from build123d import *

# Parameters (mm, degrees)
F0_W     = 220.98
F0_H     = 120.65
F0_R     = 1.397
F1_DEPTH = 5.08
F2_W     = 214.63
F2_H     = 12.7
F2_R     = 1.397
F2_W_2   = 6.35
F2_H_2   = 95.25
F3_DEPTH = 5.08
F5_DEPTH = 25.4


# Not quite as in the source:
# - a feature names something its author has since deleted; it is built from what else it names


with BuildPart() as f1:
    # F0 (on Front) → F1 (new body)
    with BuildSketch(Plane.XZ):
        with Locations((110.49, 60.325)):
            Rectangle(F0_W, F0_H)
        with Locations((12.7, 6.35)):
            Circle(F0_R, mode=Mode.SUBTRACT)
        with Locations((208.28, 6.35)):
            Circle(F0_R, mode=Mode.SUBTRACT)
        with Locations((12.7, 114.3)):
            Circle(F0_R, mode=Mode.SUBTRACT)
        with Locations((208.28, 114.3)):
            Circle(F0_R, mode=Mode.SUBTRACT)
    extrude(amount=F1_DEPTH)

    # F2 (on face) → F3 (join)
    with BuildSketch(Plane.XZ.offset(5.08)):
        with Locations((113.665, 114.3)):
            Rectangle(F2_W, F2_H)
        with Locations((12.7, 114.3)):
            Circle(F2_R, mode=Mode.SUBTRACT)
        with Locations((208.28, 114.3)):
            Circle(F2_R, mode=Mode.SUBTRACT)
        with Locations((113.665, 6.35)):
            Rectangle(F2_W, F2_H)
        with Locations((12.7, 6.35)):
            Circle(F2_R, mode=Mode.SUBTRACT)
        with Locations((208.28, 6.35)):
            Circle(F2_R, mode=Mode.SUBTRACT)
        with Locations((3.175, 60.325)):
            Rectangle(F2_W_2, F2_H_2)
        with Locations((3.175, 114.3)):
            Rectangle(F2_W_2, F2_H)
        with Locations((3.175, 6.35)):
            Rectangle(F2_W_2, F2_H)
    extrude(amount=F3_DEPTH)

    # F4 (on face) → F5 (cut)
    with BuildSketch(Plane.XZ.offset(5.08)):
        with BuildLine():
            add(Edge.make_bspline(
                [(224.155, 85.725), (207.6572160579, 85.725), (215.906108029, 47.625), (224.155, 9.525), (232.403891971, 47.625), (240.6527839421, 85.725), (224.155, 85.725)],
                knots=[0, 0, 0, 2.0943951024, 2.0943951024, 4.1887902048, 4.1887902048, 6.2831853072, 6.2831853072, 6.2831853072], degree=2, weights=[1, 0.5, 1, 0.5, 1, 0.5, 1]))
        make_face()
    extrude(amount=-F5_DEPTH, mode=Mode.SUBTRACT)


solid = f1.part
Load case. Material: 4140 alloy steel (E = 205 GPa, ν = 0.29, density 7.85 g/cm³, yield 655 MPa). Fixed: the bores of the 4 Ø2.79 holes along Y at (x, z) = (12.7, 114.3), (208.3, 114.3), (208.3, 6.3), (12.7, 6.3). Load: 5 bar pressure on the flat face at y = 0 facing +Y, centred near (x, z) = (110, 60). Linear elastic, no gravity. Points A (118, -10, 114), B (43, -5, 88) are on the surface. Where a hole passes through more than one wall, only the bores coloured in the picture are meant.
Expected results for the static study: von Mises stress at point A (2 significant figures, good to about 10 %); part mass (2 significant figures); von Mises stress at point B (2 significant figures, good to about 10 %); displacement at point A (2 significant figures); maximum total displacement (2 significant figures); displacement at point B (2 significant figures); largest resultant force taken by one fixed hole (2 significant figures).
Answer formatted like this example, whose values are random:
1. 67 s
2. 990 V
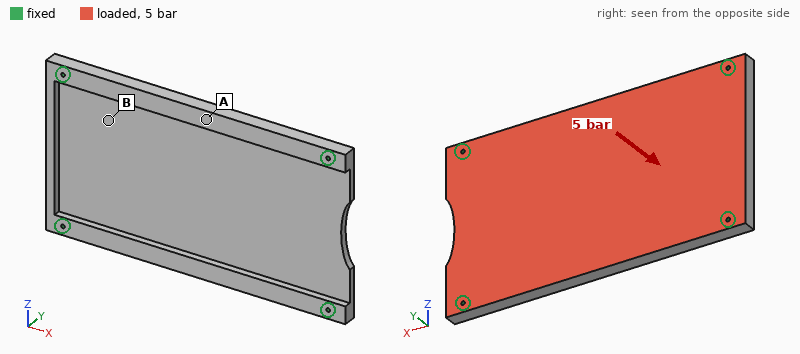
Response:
1. 160 MPa
2. 1.3 kg
3. 37 MPa
4. 0.34 mm
5. 0.48 mm
6. 0.18 mm
7. 5.0 kN
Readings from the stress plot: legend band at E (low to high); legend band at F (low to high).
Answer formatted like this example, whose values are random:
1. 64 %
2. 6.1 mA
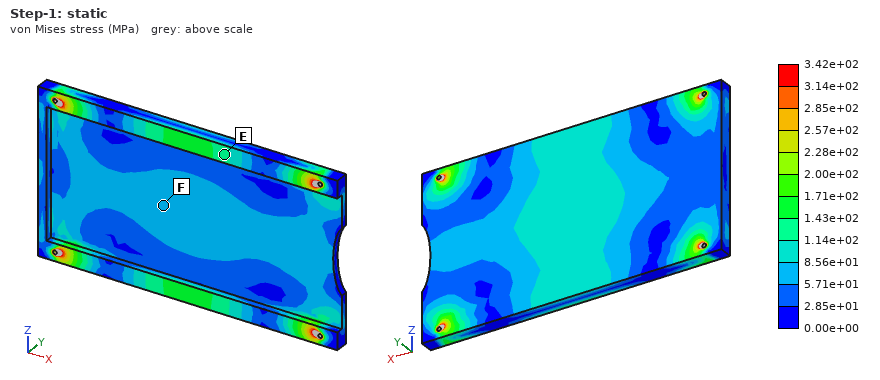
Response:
1. 1.14e+02 to 1.43e+02 MPa
2. 5.71e+01 to 8.56e+01 MPa
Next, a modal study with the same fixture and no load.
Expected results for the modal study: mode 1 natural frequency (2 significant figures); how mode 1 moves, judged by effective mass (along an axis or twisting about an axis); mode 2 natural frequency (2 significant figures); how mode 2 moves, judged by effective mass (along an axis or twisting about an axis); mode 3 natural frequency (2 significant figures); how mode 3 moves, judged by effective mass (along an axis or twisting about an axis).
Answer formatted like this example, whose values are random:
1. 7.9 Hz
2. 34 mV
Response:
1. 920 Hz
2. along Y
3. 1400 Hz
4. twisting about X
5. 2100 Hz
6. twisting about Z
